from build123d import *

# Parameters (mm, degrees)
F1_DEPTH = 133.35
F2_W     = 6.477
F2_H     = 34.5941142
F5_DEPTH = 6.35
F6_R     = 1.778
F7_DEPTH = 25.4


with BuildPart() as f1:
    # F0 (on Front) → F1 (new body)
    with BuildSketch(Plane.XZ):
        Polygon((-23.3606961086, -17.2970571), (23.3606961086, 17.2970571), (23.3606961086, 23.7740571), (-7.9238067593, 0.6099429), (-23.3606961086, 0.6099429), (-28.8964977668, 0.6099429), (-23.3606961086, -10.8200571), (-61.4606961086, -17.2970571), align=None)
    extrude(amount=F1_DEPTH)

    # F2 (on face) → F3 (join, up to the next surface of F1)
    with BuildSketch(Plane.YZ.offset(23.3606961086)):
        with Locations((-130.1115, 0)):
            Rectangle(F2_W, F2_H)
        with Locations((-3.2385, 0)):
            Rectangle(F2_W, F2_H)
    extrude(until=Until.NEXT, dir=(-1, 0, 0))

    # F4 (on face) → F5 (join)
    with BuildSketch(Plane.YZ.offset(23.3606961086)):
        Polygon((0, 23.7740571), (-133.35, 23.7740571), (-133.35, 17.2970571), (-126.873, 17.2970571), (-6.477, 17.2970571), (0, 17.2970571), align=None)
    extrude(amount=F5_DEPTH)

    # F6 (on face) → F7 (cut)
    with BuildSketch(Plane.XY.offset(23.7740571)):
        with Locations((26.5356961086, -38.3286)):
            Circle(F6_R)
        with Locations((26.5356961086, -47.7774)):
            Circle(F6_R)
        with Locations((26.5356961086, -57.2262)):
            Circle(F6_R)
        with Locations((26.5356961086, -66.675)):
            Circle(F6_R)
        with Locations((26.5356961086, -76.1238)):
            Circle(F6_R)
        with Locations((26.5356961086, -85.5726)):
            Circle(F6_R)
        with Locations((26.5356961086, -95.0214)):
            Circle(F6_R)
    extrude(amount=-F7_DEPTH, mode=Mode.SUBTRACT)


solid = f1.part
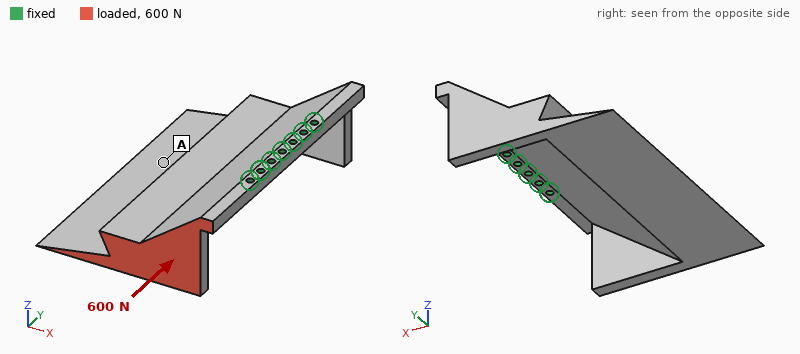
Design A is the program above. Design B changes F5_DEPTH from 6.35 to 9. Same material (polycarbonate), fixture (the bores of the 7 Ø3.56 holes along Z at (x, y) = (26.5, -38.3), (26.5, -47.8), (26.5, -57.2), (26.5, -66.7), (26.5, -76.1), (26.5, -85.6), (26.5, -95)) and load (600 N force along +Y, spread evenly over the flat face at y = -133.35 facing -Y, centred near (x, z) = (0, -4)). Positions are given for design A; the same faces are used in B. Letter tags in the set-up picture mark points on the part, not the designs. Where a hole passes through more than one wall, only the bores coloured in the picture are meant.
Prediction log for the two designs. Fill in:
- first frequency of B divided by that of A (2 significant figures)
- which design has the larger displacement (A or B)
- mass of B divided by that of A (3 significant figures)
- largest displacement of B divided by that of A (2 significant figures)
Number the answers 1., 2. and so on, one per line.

1. 1.0
2. A
3. 1.03
4. 0.91
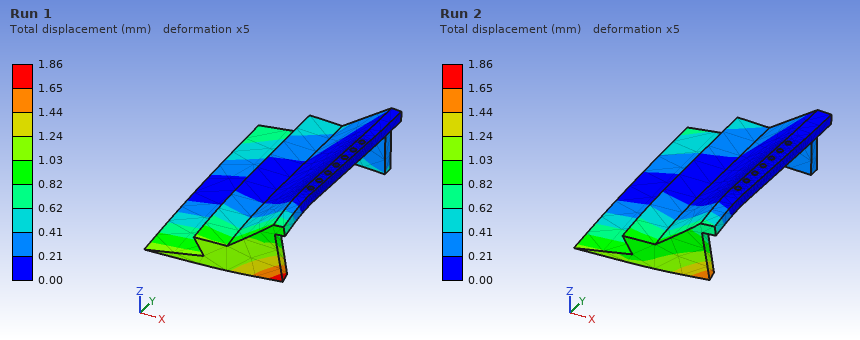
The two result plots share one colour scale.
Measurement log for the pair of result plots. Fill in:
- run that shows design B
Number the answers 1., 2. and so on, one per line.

1. Run 2
